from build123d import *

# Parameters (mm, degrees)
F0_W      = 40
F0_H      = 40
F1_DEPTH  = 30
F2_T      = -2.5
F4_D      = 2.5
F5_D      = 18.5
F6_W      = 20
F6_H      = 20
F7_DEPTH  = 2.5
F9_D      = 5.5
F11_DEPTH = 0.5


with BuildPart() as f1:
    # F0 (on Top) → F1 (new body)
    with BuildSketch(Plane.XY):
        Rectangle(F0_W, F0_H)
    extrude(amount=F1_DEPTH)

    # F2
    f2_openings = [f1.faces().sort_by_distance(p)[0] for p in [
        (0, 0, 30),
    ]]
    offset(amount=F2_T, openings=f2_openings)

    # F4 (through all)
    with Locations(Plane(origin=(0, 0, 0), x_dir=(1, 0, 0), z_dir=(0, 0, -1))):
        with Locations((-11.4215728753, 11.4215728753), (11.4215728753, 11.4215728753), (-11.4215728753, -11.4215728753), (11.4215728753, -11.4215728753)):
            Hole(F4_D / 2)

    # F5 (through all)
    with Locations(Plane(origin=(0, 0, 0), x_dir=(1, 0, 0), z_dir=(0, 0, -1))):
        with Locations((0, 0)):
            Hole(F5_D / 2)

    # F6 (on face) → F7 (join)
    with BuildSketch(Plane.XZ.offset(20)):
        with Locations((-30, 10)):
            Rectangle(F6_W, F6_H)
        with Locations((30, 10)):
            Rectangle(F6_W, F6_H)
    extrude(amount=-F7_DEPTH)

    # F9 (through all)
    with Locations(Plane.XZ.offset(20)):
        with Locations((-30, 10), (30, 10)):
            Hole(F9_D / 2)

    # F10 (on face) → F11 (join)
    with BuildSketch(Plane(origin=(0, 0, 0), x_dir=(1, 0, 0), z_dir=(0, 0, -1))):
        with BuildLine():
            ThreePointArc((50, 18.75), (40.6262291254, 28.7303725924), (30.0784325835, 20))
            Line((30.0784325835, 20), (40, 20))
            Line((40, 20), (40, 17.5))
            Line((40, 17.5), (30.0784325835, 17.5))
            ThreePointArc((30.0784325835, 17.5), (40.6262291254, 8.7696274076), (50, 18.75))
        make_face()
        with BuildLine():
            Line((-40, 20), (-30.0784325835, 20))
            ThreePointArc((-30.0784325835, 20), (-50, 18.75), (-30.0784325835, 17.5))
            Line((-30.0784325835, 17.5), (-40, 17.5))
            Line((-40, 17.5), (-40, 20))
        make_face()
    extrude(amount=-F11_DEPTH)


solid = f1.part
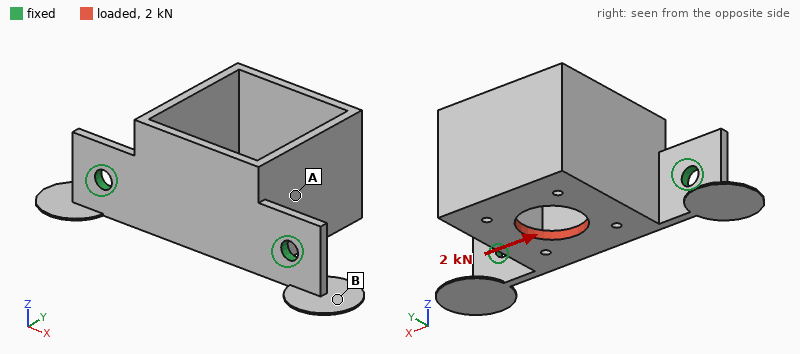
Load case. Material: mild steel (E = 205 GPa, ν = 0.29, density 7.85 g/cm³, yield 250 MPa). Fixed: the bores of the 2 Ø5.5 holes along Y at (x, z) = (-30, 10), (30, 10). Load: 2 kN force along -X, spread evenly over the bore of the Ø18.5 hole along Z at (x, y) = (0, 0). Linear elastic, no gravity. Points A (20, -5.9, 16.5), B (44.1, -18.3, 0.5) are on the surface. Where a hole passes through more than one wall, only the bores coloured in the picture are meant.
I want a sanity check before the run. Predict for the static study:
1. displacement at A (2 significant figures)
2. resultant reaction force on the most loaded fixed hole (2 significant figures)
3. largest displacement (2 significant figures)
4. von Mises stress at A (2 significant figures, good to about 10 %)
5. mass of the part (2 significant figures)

22 µm
1.3 kN
86 µm
23 MPa
120 g
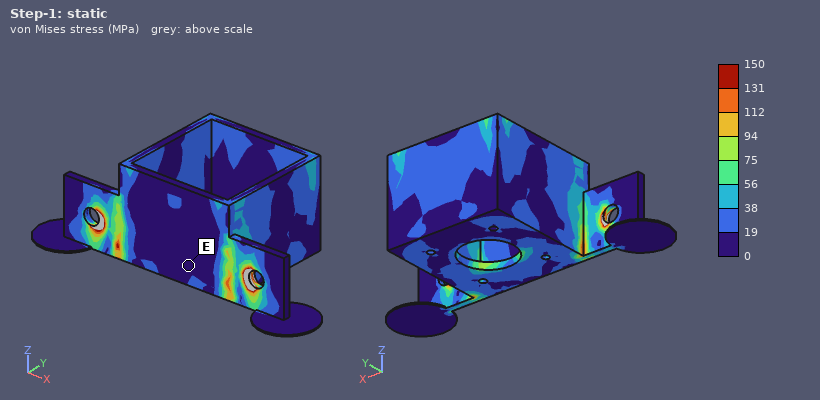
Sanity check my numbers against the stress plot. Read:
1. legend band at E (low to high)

0 to 19 MPa
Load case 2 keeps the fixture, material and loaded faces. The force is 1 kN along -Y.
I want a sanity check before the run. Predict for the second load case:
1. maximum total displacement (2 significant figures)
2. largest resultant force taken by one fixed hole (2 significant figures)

0.13 mm
560 N
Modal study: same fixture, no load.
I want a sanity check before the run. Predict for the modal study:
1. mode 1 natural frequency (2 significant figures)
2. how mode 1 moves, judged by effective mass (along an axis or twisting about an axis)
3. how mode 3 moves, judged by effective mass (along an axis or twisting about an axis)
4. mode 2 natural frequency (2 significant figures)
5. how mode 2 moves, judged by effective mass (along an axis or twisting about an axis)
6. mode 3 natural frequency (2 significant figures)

970 Hz
along Z
along Y
1900 Hz
along X
3900 Hz
